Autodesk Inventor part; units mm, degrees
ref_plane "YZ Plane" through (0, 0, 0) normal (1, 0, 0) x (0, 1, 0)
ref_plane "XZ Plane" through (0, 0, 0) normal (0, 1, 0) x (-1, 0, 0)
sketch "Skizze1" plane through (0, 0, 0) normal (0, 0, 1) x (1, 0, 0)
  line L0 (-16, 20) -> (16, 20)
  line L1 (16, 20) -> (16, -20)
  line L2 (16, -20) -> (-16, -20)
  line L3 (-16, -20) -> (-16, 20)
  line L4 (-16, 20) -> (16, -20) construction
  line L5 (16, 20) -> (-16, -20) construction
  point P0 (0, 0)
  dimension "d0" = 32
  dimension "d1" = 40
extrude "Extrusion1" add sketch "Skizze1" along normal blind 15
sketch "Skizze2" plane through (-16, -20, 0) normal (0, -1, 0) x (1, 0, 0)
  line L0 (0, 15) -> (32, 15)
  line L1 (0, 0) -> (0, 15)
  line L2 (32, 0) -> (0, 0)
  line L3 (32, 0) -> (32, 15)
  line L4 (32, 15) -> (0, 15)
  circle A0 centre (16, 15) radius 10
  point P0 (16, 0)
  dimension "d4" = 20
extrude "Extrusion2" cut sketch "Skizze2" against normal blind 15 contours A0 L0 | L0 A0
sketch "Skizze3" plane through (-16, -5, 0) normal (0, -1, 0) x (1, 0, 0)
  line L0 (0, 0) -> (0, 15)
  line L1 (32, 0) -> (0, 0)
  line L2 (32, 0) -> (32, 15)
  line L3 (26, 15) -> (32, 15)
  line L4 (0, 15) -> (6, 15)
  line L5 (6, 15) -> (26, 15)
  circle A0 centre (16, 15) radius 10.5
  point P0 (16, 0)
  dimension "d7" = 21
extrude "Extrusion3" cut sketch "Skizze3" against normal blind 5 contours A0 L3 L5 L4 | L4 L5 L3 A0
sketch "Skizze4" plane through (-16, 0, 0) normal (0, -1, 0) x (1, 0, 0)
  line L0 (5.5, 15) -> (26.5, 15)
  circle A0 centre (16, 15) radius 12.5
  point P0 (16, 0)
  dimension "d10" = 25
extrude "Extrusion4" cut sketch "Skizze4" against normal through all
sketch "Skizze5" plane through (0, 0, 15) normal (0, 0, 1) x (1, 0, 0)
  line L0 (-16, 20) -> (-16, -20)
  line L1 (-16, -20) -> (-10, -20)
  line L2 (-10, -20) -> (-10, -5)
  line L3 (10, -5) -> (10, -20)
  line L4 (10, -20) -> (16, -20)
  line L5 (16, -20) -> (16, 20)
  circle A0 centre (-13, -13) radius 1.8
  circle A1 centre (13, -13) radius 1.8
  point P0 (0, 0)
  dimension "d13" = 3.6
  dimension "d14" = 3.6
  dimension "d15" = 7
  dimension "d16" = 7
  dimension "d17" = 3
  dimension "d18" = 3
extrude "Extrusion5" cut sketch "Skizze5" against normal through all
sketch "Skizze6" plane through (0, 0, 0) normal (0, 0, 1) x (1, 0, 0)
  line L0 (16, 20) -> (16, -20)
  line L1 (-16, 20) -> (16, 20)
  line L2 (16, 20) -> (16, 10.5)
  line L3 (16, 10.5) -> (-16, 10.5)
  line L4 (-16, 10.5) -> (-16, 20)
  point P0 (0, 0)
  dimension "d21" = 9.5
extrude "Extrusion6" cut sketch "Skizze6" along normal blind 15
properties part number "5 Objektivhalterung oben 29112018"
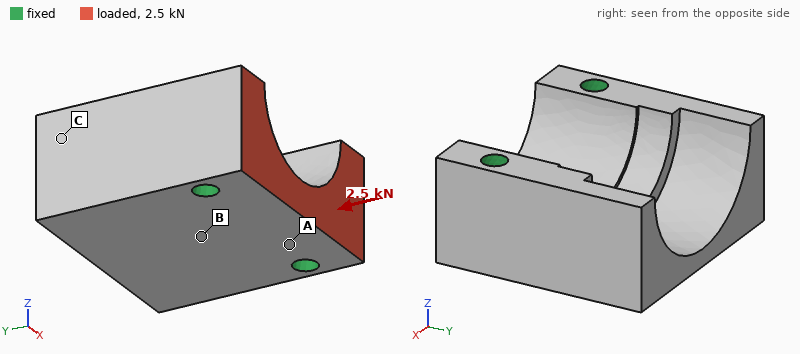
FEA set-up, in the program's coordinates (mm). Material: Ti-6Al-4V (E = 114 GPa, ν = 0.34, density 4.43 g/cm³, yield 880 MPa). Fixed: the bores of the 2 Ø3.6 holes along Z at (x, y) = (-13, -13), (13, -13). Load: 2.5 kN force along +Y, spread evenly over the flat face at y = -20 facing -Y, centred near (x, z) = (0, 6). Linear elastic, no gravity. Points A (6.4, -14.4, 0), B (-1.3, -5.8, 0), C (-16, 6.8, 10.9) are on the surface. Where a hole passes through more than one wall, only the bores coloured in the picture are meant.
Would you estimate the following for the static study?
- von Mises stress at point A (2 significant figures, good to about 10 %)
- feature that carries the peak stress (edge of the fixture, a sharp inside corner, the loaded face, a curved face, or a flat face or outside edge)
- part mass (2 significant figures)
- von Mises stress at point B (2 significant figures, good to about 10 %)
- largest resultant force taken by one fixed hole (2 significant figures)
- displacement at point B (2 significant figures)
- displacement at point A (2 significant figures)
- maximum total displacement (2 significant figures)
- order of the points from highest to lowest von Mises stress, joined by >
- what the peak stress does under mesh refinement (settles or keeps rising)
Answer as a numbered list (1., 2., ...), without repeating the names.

1. 7.0 MPa
2. edge of the fixture
3. 38 g
4. 3.9 MPa
5. 1.3 kN
6. 0.96 µm
7. 0.97 µm
8. 1.7 µm
9. A > B > C
10. keeps rising
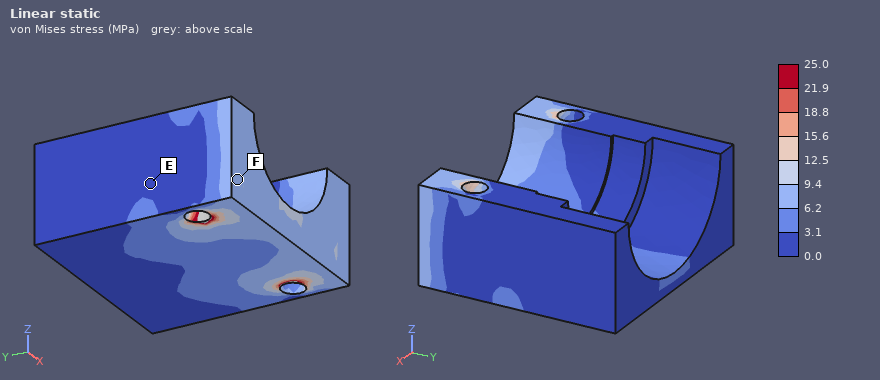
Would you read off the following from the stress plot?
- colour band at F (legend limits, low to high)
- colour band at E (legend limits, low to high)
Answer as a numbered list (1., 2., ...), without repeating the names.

1. 6.2 to 9.4 MPa
2. 0.0 to 3.1 MPa
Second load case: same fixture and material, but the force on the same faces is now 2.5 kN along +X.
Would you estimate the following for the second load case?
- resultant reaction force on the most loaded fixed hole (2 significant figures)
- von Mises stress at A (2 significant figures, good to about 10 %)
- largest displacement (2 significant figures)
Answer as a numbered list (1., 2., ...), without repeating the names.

1. 1.3 kN
2. 13 MPa
3. 3.1 µm
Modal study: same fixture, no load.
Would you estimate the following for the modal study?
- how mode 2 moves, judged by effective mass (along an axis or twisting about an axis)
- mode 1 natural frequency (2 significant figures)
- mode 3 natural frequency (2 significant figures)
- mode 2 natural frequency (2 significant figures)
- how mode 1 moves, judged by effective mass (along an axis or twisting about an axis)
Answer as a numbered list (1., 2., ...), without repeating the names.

1. along X
2. 18 kHz
3. 22 kHz
4. 18 kHz
5. along Z
